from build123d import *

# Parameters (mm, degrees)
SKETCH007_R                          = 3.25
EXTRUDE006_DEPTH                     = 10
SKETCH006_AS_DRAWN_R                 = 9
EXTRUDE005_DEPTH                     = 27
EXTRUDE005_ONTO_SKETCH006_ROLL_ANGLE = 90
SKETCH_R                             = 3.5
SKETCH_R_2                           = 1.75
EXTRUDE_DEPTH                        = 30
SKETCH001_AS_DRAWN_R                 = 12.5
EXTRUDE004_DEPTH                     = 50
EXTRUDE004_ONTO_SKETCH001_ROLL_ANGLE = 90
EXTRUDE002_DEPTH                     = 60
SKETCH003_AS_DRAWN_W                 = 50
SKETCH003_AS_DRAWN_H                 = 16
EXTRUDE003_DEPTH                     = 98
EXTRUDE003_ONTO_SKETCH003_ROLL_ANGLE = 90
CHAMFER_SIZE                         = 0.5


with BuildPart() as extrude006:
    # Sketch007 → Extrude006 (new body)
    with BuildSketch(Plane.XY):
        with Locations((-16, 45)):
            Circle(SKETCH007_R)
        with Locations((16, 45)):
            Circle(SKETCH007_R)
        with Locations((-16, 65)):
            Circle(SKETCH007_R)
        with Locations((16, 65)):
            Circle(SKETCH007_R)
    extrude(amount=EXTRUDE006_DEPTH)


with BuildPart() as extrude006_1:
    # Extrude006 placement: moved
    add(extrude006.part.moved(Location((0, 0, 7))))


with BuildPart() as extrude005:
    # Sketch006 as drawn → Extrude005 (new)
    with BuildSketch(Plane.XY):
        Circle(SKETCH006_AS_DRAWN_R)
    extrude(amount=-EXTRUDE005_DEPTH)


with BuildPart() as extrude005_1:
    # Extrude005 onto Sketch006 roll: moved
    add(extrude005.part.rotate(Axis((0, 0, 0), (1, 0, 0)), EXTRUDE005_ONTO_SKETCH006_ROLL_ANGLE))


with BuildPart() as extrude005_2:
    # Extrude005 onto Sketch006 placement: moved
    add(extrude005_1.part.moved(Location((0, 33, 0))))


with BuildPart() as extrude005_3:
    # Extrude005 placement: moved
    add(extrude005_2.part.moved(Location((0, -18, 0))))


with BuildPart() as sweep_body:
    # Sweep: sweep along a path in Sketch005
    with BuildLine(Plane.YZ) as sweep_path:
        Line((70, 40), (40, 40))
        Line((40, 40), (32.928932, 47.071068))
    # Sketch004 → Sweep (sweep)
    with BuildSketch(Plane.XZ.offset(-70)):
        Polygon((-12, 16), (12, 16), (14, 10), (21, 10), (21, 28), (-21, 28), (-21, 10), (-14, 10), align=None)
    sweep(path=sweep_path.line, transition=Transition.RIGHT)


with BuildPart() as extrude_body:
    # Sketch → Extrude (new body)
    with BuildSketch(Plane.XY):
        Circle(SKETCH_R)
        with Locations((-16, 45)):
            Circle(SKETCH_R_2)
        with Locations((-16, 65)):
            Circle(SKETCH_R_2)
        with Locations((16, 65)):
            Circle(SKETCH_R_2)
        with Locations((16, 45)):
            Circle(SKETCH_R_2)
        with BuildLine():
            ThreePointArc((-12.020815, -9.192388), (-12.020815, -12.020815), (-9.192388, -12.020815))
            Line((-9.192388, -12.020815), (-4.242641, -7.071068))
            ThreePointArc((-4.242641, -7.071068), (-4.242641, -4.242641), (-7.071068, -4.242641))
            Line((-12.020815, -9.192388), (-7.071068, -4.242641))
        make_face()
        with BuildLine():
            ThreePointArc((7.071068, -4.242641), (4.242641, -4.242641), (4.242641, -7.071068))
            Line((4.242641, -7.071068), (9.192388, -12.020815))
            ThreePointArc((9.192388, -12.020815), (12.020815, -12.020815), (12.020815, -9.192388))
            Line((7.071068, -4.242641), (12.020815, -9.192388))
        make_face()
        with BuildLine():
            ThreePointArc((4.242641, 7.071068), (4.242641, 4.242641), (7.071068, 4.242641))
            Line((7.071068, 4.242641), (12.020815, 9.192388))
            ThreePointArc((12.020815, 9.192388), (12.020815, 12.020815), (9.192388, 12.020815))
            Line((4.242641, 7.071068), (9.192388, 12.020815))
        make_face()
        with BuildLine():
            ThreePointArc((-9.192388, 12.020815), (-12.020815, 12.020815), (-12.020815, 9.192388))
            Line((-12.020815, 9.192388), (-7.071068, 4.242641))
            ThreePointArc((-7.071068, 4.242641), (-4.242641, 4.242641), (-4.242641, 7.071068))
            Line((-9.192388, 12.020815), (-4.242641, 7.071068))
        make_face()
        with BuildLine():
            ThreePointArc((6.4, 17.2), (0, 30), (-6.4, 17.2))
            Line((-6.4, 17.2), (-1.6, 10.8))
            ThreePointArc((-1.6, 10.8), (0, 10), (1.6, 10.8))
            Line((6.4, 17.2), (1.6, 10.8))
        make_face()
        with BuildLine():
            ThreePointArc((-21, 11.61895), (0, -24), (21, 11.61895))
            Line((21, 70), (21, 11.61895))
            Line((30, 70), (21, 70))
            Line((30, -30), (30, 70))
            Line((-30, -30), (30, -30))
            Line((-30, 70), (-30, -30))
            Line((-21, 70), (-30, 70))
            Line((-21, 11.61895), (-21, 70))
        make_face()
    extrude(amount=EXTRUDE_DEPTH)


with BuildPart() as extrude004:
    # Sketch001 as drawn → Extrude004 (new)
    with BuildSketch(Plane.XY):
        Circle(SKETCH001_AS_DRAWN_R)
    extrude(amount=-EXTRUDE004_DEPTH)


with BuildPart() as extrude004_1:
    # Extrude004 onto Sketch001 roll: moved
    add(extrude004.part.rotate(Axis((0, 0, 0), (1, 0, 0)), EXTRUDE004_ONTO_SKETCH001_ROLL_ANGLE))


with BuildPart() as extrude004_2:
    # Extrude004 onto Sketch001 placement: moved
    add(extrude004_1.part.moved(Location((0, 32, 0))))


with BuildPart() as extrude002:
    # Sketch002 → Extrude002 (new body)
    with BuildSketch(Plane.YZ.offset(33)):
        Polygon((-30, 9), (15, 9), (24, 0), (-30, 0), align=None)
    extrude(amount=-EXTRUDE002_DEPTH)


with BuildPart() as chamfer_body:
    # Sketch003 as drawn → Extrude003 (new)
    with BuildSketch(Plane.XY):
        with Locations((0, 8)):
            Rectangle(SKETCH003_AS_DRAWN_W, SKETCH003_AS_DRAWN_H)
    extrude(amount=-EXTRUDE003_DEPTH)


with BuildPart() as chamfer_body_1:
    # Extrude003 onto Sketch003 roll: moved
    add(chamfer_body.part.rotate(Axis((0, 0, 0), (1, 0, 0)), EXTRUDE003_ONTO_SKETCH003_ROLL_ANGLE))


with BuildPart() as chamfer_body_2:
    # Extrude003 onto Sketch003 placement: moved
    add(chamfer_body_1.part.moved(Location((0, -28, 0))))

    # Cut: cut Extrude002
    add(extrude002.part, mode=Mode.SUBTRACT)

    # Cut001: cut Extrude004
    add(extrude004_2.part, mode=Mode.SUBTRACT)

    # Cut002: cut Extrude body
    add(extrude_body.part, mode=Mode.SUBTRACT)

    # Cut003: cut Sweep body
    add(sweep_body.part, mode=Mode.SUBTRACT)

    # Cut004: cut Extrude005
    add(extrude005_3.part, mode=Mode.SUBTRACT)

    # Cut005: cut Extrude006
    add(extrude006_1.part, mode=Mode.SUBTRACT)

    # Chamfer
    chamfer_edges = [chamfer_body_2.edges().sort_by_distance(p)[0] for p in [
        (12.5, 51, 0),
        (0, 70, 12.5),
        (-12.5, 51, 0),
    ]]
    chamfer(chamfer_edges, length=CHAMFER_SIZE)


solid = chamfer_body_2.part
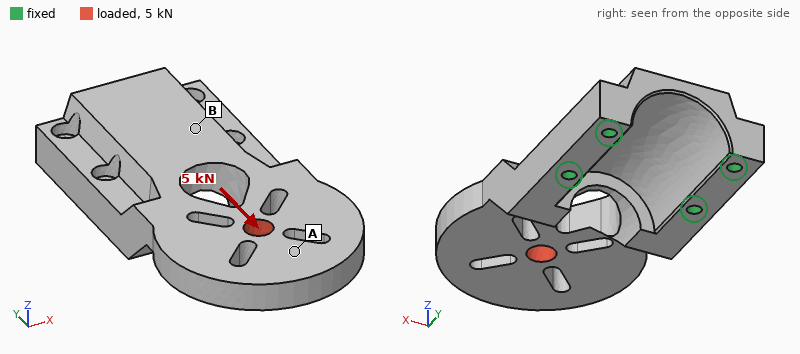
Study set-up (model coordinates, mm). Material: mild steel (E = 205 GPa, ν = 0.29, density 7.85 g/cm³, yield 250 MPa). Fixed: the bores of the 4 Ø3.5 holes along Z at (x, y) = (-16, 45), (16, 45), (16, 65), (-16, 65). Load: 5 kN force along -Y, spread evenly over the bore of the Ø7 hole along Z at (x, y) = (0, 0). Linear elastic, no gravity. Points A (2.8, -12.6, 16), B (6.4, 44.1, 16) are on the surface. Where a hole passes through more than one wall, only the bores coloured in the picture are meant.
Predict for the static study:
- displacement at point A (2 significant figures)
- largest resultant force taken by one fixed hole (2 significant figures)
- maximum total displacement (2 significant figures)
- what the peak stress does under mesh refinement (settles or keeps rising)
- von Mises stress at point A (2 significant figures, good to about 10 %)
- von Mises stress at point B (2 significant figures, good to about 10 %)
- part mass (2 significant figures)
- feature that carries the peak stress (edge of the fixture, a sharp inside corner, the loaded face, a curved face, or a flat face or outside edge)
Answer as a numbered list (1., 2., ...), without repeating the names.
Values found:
1. 49 µm
2. 1.7 kN
3. 60 µm
4. keeps rising
5. 12 MPa
6. 31 MPa
7. 210 g
8. edge of the fixture
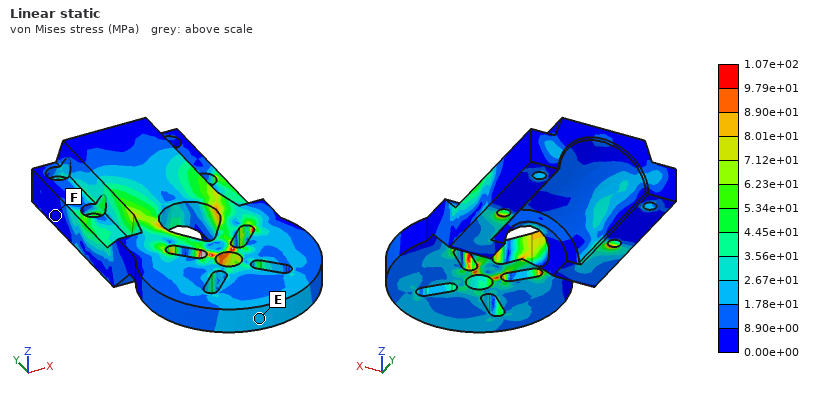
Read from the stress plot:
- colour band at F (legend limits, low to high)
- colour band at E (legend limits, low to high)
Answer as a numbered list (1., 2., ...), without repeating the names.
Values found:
1. 0.00e+00 to 8.90e+00 MPa
2. 1.78e+01 to 2.67e+01 MPa
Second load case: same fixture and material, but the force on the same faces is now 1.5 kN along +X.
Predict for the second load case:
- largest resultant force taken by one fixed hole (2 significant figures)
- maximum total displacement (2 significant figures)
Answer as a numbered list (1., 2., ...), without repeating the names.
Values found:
1. 1.7 kN
2. 27 µm
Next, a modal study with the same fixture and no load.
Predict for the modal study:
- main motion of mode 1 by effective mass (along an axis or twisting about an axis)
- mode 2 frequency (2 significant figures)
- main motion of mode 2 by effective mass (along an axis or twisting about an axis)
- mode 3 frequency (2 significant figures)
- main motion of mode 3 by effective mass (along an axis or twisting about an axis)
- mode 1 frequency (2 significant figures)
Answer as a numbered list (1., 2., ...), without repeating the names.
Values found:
1. along Z
2. 3900 Hz
3. along X
4. 6000 Hz
5. along X
6. 2000 Hz
